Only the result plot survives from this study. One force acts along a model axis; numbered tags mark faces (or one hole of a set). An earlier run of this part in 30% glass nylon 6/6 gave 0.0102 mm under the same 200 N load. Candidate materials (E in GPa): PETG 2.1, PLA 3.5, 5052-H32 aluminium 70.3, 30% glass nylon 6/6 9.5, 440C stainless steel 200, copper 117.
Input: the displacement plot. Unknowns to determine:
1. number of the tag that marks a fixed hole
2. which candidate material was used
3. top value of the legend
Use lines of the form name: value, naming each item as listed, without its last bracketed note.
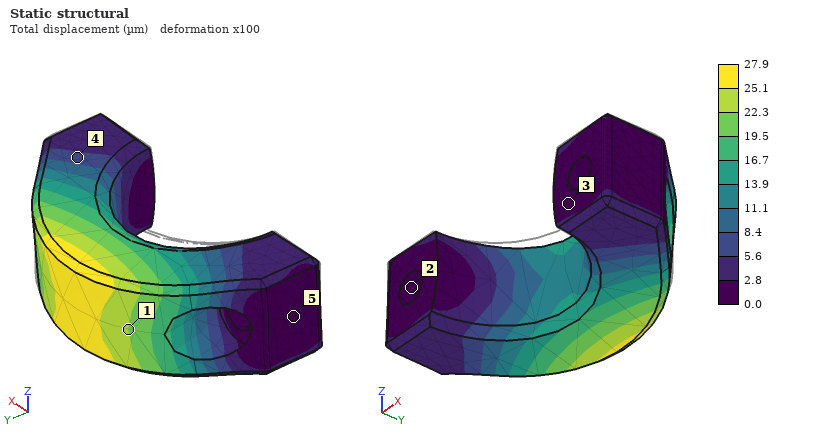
number of the tag that marks a fixed hole: 2
which candidate material was used: PLA
top value of the legend: 27.9 µm
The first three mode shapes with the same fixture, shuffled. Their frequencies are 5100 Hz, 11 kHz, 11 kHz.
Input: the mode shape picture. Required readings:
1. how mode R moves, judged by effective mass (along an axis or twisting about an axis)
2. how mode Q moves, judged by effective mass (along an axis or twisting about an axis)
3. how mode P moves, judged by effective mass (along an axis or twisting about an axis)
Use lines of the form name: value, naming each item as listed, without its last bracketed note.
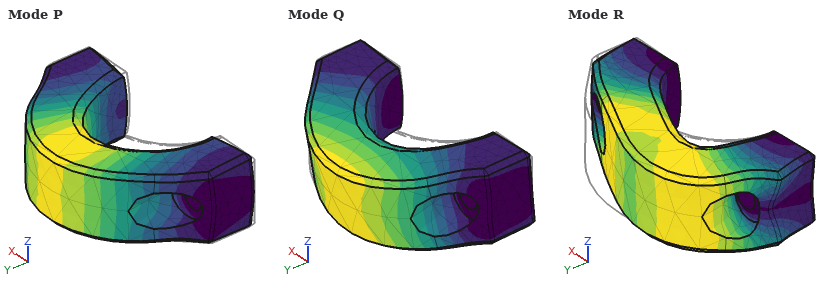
how mode R moves, judged by effective mass: along X
how mode Q moves, judged by effective mass: along Z
how mode P moves, judged by effective mass: along Y
